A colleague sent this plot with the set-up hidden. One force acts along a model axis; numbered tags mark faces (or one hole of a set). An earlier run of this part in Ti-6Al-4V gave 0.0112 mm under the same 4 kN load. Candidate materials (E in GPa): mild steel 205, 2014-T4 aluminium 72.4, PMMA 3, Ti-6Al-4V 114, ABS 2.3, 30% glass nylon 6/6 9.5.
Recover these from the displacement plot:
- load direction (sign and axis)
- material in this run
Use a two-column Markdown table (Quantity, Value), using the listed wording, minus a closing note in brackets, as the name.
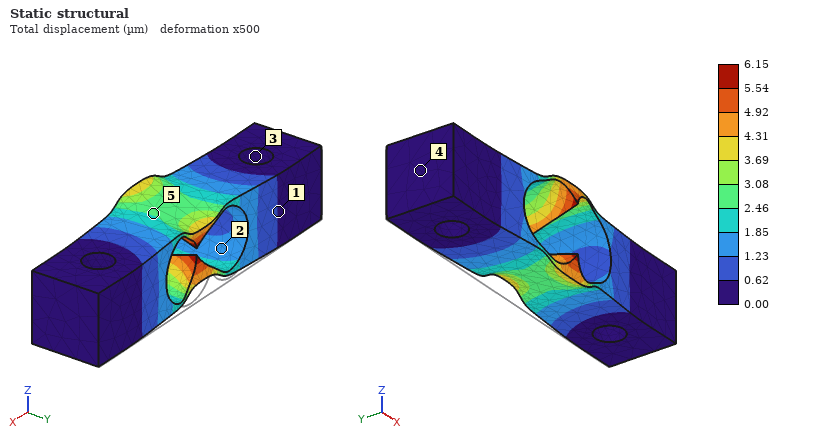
| Quantity | Value |
|---|---|
| load direction | -Y |
| material in this run | mild steel |
